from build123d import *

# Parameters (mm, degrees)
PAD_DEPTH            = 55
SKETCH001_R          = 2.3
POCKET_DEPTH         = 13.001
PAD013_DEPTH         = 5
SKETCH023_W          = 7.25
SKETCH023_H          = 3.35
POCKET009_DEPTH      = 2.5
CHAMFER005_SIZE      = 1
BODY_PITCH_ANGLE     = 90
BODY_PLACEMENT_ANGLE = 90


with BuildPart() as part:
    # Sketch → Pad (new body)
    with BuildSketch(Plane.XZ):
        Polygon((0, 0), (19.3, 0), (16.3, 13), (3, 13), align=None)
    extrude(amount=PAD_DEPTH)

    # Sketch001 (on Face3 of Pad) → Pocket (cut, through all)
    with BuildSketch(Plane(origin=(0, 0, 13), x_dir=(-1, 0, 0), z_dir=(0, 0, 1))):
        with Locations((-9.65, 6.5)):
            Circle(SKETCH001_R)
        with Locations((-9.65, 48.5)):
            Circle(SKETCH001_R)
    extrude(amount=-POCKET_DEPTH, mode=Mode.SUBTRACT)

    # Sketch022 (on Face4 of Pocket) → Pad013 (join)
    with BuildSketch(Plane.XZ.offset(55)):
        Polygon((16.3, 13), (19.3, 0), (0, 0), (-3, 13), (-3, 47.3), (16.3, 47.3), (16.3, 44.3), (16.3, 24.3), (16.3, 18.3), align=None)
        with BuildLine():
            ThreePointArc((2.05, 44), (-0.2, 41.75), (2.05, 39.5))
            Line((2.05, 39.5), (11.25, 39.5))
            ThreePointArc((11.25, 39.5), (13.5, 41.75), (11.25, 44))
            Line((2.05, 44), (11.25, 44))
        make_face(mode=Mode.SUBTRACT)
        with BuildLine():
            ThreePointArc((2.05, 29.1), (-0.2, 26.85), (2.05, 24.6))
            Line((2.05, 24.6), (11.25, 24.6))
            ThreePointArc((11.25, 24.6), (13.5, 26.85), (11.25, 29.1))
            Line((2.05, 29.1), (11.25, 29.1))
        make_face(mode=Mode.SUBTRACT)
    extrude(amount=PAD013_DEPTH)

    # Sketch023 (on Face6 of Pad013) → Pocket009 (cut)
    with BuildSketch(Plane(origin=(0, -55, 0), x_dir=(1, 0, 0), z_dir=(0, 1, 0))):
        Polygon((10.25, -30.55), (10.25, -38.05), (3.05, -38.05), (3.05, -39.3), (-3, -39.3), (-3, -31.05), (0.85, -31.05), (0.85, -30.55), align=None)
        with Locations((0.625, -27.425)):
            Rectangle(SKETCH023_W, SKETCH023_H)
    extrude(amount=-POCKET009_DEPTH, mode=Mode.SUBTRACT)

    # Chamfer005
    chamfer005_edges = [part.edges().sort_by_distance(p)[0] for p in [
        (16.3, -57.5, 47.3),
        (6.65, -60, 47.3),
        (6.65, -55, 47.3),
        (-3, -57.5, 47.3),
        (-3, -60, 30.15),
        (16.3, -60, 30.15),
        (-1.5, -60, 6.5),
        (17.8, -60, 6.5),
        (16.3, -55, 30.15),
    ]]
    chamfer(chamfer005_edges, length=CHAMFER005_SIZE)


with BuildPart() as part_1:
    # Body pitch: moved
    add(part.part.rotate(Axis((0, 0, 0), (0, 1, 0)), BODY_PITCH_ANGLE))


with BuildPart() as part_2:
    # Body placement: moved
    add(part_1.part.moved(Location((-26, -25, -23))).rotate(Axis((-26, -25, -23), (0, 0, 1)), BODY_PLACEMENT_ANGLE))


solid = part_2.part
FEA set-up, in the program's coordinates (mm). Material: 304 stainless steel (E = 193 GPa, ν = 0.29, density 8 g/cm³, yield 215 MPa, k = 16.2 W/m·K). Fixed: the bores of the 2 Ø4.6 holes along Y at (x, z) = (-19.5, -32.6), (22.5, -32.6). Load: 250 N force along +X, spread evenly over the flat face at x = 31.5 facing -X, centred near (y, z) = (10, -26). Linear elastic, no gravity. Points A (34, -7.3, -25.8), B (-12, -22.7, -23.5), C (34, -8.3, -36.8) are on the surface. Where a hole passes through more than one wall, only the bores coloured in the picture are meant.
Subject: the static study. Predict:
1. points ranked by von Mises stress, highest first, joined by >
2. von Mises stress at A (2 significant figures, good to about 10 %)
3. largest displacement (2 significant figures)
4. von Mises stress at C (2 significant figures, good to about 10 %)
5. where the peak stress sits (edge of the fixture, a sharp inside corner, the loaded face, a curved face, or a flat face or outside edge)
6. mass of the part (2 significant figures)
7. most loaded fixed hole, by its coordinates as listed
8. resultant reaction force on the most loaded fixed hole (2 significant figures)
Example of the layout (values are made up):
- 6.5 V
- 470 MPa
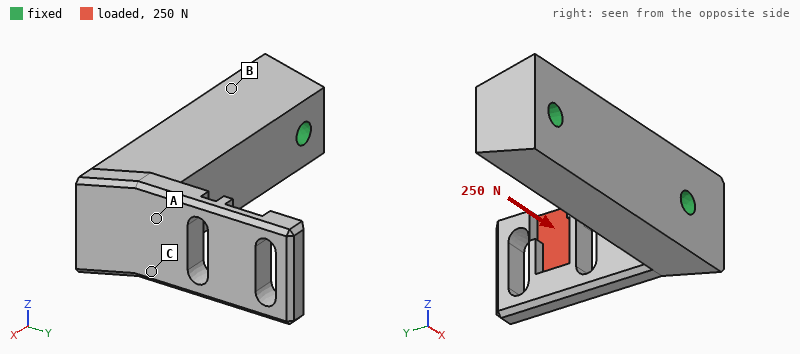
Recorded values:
- C > A > B
- 46 MPa
- 0.13 mm
- 67 MPa
- a curved face
- 120 g
- (22.5, -32.6)
- 260 N
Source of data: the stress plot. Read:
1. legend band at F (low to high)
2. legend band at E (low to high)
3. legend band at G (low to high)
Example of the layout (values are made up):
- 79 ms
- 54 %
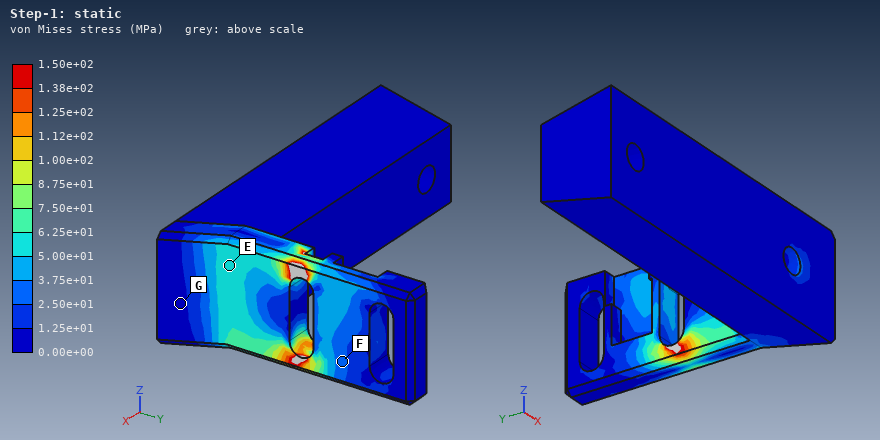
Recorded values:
- 2.50e+01 to 3.75e+01 MPa
- 5.00e+01 to 6.25e+01 MPa
- 0.00e+00 to 1.25e+01 MPa
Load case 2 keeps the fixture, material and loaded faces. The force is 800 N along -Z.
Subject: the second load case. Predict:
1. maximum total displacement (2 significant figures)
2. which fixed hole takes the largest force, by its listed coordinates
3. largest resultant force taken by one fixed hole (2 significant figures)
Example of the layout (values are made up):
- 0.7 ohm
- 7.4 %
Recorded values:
- 57 µm
- (22.5, -32.6)
- 880 N
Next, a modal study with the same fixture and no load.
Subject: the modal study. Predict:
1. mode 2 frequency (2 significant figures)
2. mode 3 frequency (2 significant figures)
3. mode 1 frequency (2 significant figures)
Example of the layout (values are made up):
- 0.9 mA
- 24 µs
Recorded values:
- 6300 Hz
- 8000 Hz
- 2500 Hz
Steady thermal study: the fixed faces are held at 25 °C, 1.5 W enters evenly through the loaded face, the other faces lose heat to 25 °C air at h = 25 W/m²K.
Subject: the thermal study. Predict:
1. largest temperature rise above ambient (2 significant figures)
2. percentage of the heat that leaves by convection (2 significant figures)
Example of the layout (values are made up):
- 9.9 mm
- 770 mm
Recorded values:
- 33 K
- 56 %
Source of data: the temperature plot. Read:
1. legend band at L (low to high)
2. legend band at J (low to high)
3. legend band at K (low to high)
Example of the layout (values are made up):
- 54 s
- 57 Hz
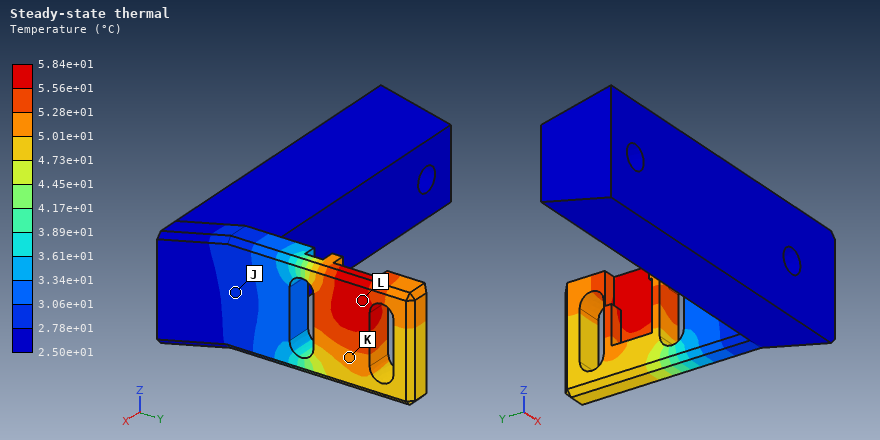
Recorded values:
- 5.56e+01 to 5.84e+01 °C
- 2.78e+01 to 3.06e+01 °C
- 5.01e+01 to 5.28e+01 °C
